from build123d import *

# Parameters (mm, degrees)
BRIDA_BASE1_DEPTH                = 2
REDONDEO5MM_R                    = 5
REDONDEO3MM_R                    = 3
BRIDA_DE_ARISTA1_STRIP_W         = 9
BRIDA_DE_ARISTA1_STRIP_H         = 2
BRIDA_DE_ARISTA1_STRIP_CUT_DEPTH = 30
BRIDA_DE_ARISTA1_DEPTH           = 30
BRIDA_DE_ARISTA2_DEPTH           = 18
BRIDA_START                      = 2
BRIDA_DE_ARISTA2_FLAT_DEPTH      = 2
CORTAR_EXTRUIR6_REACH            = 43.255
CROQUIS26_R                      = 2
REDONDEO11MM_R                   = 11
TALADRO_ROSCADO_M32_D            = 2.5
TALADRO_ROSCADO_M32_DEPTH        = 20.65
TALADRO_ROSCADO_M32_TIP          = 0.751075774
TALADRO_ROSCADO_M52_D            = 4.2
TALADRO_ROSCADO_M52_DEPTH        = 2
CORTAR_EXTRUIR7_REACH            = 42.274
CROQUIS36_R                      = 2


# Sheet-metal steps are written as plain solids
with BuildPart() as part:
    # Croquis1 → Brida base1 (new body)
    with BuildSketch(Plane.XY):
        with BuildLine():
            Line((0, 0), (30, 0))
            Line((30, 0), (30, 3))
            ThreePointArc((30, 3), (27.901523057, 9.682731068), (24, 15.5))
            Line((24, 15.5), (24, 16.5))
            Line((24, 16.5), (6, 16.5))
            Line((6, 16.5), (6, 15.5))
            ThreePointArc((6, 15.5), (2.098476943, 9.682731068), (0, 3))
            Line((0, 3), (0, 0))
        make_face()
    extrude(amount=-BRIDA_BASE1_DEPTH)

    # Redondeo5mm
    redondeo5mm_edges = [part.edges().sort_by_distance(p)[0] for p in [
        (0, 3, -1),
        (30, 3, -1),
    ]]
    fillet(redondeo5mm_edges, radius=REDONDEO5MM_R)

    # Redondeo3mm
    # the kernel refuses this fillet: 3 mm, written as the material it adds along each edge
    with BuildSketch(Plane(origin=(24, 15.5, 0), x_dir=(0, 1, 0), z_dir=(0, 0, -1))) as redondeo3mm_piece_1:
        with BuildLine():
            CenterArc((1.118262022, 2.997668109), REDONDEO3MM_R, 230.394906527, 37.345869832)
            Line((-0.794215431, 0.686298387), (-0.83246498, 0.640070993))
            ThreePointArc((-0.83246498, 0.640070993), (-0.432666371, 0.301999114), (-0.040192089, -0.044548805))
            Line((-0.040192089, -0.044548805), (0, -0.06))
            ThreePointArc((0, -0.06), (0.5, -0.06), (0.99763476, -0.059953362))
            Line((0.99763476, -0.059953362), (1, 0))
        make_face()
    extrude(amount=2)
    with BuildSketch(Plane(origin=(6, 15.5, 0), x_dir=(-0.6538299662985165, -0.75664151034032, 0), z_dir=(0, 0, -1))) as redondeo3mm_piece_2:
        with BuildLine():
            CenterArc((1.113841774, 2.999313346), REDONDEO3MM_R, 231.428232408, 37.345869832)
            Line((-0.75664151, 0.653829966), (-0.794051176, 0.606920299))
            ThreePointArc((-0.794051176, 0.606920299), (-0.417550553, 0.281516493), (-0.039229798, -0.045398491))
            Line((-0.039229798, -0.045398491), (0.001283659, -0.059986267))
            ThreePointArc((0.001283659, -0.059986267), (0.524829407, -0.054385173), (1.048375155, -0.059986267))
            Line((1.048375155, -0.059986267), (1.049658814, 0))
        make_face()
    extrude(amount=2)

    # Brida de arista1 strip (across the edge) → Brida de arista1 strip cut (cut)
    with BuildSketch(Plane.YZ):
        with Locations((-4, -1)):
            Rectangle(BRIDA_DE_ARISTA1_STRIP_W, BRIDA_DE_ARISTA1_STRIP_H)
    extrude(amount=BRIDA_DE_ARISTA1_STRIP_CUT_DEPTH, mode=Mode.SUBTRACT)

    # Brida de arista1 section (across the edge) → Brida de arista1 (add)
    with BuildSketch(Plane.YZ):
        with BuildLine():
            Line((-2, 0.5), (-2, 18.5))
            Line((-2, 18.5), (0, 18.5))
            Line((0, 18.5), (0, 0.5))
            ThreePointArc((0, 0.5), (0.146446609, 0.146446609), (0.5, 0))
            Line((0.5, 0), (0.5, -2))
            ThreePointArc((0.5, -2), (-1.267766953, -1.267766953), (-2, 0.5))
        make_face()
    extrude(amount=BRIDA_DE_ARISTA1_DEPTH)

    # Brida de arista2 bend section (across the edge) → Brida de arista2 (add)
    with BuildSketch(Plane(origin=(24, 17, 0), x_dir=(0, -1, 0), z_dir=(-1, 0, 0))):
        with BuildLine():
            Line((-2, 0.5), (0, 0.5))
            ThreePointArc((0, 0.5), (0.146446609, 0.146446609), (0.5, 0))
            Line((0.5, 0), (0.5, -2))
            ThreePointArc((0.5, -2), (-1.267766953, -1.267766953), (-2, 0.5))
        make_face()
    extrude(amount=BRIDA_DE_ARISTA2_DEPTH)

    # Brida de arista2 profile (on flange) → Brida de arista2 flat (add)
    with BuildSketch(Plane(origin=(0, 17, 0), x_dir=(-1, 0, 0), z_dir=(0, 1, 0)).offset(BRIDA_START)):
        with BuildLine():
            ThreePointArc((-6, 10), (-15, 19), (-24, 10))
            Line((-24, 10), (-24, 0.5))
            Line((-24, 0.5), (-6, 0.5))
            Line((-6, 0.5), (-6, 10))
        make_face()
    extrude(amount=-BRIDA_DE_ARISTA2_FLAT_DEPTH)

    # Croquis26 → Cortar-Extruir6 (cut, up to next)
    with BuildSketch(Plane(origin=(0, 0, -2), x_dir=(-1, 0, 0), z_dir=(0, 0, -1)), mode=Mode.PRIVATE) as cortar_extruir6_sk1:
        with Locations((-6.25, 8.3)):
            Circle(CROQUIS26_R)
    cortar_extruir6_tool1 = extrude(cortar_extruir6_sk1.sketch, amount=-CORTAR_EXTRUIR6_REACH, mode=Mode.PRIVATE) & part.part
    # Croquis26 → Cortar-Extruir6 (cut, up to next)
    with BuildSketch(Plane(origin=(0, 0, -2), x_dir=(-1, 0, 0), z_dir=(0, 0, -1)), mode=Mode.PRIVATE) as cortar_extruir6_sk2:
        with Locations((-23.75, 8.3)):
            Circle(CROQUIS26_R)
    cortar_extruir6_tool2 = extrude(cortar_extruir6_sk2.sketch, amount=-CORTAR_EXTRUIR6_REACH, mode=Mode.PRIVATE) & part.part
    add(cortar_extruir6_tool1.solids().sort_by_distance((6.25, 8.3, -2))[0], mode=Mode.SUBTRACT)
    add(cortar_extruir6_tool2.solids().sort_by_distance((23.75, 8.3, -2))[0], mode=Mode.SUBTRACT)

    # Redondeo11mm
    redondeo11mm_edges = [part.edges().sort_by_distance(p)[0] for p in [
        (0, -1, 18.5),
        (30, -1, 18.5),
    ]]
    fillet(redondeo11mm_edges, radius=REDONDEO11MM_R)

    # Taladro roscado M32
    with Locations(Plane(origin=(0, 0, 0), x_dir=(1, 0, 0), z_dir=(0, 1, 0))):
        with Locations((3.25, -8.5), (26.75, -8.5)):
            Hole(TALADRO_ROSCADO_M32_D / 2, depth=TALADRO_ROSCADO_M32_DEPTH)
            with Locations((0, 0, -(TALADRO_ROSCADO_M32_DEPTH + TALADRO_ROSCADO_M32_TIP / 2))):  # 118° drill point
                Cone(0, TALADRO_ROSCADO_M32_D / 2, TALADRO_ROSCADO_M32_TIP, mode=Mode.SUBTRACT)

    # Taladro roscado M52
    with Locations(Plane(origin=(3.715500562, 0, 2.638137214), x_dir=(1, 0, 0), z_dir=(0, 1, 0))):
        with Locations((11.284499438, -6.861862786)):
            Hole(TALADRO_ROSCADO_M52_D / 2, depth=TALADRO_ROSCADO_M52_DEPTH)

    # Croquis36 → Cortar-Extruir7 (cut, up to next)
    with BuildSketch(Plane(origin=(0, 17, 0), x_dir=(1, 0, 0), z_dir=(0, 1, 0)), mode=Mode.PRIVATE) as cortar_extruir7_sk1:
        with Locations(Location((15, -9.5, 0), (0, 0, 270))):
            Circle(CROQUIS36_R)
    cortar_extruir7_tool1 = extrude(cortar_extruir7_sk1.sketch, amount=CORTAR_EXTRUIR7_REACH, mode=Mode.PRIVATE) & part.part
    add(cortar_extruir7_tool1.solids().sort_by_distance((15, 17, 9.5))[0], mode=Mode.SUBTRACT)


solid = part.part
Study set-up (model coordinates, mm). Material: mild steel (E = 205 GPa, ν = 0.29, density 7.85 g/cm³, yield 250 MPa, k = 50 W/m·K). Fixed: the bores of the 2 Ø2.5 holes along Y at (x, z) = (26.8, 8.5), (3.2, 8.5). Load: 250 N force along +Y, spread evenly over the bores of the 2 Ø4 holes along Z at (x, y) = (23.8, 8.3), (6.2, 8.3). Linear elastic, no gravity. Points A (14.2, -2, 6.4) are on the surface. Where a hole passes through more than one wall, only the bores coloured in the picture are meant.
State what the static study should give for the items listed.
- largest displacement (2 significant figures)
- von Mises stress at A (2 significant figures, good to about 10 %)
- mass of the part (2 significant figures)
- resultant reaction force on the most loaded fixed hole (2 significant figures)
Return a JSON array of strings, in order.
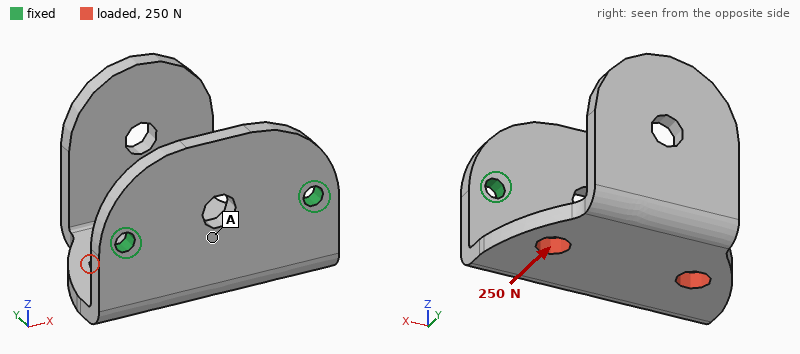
["73 µm", "24 MPa", "20 g", "130 N"]
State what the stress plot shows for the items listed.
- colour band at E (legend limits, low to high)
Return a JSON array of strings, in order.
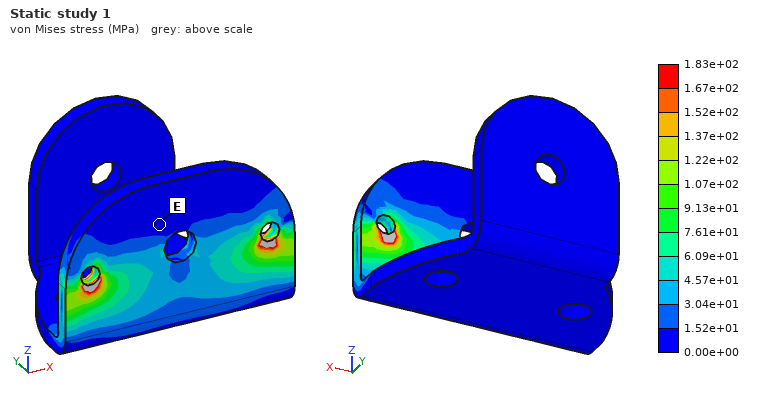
["0.00e+00 to 1.52e+01 MPa"]
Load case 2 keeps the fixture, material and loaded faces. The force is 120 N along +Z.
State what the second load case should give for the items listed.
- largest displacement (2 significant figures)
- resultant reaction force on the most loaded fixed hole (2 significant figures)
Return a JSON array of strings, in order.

["95 µm", "61 N"]
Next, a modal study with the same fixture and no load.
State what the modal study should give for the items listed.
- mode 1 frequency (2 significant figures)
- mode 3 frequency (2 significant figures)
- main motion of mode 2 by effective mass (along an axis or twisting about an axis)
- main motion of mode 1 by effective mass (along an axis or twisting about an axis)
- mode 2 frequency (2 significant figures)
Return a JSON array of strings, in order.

["1400 Hz", "3300 Hz", "along X", "along Z", "2700 Hz"]
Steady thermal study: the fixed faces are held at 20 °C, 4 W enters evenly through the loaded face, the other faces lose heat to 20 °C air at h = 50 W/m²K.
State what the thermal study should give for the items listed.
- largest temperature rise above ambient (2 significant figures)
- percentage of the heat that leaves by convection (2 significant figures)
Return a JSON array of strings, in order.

["22 K", "38 %"]
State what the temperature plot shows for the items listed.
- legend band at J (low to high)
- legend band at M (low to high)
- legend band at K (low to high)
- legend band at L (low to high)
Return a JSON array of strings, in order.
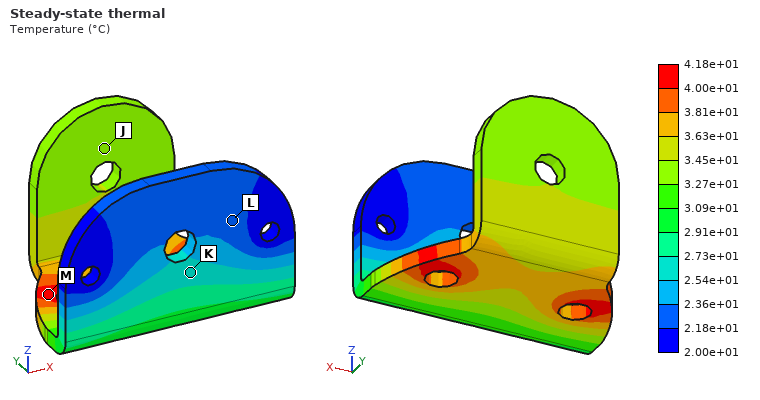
["3.27e+01 to 3.45e+01 °C", "4.00e+01 to 4.18e+01 °C", "2.54e+01 to 2.73e+01 °C", "2.18e+01 to 2.36e+01 °C"]
